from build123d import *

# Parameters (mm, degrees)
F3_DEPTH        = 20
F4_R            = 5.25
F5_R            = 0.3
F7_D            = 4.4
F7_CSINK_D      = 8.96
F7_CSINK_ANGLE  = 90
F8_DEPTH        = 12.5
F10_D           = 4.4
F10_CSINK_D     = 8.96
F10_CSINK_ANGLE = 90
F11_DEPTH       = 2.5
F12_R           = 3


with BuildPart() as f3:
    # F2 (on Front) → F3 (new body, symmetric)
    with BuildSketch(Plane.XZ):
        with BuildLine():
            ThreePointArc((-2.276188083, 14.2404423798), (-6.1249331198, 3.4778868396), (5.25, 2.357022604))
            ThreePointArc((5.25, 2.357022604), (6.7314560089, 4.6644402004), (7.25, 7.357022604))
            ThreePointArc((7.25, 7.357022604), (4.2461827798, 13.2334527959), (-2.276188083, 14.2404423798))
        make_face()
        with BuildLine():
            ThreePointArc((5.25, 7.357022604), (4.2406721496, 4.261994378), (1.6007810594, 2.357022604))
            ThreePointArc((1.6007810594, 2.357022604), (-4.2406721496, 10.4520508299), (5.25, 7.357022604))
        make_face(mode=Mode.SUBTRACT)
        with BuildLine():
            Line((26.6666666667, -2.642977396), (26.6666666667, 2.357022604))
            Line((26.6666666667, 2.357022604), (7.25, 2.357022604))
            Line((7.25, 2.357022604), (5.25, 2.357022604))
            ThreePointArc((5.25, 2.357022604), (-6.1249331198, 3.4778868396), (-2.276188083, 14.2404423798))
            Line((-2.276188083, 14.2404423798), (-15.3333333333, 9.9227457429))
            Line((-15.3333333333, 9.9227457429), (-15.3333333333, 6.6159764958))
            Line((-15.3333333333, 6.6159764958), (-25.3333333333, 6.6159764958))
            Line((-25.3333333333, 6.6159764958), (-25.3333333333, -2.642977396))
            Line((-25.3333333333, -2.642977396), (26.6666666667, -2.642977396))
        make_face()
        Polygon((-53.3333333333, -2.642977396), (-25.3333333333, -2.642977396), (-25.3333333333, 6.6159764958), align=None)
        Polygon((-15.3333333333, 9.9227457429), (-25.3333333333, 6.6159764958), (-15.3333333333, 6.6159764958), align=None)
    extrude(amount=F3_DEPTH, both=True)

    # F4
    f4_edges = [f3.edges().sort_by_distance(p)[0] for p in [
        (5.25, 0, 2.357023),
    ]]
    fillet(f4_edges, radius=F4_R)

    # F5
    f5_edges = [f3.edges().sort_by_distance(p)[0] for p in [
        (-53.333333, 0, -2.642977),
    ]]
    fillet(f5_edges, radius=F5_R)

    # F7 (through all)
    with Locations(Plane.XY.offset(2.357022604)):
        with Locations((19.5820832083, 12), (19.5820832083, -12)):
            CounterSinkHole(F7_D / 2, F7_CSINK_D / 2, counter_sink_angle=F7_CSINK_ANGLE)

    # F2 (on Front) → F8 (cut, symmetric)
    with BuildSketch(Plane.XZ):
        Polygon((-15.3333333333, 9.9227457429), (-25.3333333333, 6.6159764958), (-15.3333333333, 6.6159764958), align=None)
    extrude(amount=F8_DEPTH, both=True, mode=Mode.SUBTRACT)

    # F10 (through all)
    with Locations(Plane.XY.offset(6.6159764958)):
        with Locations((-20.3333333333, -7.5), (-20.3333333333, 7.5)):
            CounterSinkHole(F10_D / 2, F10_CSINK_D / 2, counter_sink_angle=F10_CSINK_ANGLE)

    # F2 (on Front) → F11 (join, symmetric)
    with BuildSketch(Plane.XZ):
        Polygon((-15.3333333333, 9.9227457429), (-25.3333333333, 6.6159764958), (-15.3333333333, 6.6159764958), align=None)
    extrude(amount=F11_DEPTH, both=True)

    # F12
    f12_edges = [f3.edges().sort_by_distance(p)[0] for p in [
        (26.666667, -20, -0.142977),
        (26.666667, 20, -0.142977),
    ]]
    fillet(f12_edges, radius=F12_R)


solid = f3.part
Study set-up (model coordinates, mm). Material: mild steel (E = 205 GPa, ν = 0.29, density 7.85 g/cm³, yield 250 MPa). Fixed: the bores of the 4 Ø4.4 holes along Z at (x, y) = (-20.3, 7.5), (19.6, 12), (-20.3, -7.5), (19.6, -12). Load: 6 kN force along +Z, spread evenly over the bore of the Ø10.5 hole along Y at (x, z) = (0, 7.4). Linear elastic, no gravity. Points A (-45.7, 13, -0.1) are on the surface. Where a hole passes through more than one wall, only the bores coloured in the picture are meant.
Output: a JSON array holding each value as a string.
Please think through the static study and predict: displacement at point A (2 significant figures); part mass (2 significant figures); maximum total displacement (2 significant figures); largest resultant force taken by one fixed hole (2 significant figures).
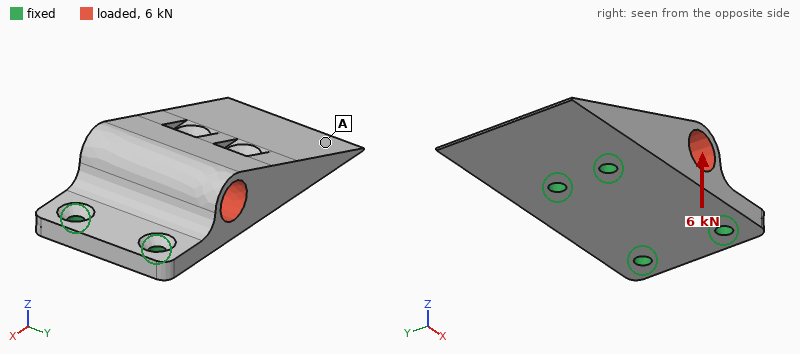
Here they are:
["6.3 µm", "180 g", "12 µm", "1.8 kN"]
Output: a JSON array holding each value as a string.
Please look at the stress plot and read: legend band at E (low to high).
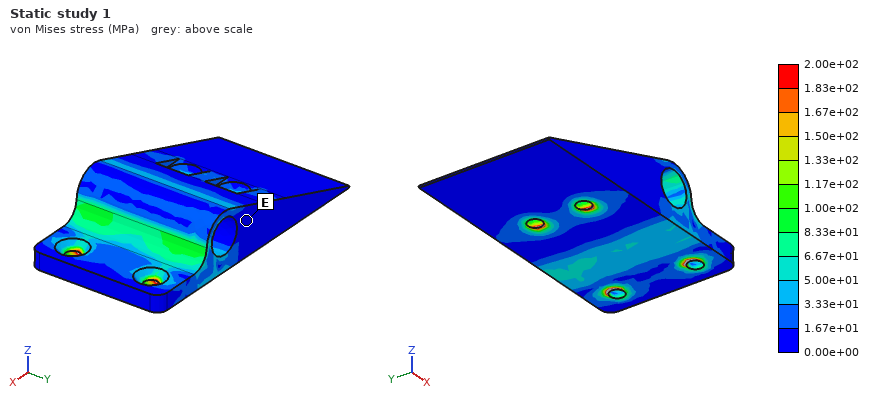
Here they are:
["0.00e+00 to 1.67e+01 MPa"]
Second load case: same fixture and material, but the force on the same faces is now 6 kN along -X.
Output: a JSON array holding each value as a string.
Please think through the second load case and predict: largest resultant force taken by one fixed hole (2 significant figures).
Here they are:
["2.1 kN"]
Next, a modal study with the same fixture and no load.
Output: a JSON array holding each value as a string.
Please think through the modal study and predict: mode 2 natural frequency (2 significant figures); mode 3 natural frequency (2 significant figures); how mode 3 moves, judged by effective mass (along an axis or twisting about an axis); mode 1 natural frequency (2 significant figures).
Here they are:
["14 kHz", "15 kHz", "along Z", "10 kHz"]
